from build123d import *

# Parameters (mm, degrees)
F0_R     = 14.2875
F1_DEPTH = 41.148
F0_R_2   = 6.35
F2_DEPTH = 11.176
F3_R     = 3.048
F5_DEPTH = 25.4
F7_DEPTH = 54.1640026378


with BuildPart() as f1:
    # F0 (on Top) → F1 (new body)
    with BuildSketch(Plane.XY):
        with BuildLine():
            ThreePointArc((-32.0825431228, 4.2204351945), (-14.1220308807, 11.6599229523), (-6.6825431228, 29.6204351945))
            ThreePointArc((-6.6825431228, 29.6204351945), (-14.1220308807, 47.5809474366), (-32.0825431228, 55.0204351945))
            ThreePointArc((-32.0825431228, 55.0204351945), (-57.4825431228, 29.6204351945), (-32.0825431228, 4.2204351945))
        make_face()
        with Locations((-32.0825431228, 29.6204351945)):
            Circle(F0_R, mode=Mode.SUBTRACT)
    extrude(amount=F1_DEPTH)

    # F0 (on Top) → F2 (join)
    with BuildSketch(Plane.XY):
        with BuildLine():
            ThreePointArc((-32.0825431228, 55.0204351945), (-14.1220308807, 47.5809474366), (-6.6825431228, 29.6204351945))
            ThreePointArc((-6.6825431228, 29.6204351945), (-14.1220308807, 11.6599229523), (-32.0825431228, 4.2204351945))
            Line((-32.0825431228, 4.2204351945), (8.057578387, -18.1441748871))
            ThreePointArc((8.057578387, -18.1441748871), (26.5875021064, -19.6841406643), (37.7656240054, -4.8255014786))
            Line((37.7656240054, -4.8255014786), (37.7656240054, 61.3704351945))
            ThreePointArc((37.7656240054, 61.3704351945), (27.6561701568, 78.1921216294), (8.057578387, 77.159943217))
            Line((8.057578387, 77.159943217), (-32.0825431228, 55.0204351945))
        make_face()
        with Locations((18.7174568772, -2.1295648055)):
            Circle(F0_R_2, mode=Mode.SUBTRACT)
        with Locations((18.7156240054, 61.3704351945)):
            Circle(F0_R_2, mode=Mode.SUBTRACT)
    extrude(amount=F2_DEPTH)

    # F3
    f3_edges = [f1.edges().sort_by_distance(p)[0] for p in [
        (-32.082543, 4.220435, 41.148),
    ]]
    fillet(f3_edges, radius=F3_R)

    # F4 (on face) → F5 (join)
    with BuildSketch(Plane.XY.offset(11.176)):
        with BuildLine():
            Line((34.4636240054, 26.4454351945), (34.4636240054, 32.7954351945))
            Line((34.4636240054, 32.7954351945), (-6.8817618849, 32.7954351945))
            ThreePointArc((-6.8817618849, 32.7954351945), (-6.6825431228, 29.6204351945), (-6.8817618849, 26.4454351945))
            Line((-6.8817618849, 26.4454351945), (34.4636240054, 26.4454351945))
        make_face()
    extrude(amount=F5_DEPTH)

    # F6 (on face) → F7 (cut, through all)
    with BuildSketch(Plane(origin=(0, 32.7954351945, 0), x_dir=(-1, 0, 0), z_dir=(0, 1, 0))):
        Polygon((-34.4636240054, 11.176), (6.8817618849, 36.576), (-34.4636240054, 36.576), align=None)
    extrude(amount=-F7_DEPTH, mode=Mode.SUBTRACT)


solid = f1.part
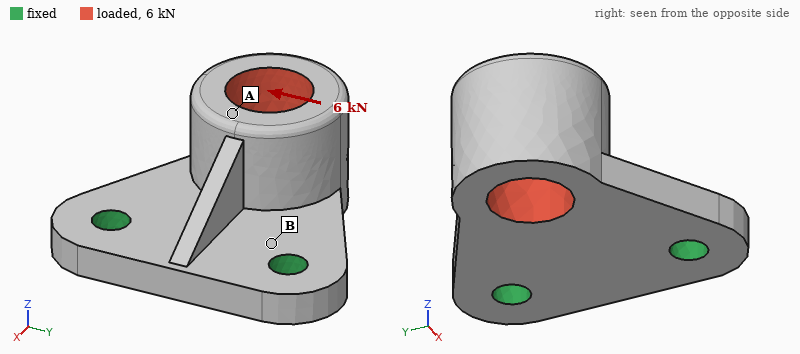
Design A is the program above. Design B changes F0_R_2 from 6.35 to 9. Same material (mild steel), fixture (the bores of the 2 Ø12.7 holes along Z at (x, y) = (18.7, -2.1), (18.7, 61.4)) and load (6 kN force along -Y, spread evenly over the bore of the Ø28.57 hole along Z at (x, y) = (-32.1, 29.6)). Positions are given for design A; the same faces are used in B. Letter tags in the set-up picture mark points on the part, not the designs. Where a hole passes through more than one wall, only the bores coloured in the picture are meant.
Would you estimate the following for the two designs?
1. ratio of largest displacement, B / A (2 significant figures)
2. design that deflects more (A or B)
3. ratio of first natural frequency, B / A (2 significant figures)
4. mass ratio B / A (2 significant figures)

0.90
A
1.1
0.97
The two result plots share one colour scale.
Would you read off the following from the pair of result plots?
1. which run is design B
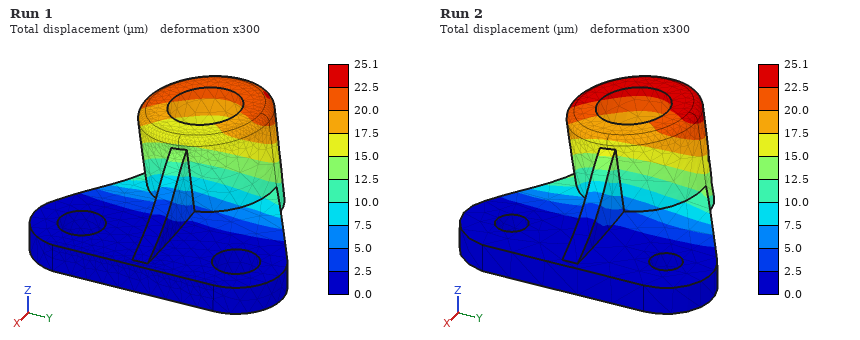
Run 1
